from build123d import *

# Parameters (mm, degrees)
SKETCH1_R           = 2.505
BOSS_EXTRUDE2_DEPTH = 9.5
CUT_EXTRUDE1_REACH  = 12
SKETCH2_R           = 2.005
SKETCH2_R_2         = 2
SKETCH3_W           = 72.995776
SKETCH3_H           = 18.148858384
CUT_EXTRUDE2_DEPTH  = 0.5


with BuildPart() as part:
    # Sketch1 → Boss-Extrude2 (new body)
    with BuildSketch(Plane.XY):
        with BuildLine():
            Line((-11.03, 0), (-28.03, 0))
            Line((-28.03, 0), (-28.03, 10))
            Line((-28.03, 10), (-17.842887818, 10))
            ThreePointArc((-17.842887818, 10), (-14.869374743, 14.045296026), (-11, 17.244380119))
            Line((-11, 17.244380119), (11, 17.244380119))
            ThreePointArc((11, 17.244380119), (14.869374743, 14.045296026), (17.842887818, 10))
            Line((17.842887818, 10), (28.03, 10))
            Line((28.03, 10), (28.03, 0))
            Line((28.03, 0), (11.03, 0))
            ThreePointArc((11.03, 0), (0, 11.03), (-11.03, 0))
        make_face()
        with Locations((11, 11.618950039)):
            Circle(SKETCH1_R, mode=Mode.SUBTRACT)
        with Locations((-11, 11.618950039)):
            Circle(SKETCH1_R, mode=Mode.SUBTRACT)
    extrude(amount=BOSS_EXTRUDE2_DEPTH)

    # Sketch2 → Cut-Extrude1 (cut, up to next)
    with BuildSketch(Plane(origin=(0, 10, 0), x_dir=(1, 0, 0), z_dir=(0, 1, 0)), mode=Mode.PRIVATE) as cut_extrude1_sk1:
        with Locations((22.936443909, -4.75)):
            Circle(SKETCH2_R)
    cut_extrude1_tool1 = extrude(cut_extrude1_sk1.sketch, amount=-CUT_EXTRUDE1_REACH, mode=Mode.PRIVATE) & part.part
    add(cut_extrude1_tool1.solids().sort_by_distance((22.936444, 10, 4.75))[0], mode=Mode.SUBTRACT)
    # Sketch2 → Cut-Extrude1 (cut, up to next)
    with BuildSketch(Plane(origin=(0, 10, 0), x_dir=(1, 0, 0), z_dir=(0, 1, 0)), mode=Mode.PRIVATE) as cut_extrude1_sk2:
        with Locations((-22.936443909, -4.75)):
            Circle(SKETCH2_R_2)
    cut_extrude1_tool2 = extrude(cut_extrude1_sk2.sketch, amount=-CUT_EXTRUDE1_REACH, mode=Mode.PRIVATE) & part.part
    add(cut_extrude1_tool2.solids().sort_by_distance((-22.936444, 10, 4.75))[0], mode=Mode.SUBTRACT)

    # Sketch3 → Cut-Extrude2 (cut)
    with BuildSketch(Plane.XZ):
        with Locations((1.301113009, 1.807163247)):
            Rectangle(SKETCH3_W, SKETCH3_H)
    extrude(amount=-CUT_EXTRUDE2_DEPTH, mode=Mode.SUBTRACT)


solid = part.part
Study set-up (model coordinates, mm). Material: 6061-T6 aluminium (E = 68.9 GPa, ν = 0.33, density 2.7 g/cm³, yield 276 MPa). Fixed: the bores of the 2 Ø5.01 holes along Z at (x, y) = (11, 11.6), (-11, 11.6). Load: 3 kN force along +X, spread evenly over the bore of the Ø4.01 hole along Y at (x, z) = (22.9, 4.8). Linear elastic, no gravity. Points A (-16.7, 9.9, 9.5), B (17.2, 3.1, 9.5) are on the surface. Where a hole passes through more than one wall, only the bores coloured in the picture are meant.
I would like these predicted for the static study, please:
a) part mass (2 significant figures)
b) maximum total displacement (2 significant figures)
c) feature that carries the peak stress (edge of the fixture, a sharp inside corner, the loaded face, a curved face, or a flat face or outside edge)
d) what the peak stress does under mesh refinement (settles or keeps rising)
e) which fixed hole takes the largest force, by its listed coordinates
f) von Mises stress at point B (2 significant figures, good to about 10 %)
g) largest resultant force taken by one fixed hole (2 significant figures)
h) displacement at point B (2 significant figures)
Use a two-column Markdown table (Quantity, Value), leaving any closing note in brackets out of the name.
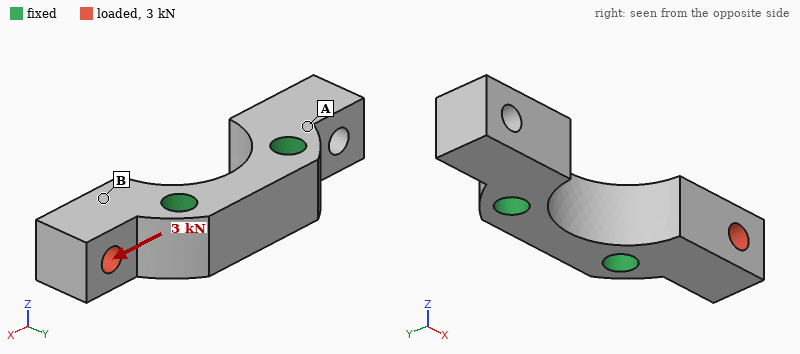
| Quantity | Value |
|---|---|
| part mass | 13 g |
| maximum total displacement | 46 µm |
| feature that carries the peak stress | edge of the fixture |
| what the peak stress does under mesh refinement | keeps rising |
| which fixed hole takes the largest force, by its listed coordinates | (11, 11.6) |
| von Mises stress at point B | 39 MPa |
| largest resultant force taken by one fixed hole | 3.0 kN |
| displacement at point B | 22 µm |
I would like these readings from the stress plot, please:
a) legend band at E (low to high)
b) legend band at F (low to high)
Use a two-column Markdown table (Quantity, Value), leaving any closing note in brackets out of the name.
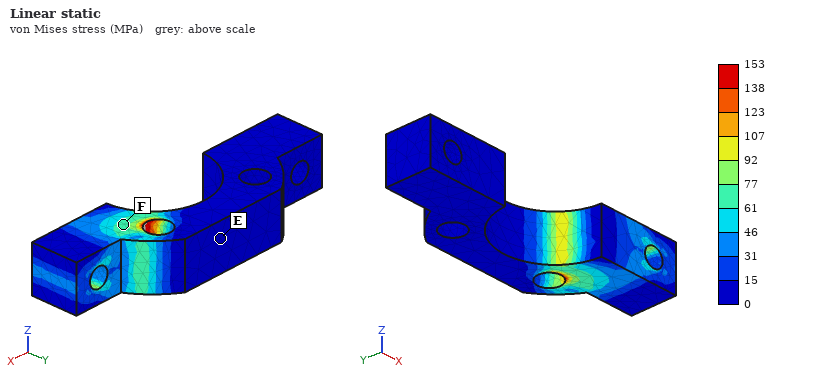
| Quantity | Value |
|---|---|
| legend band at E | 0 to 15 MPa |
| legend band at F | 61 to 77 MPa |
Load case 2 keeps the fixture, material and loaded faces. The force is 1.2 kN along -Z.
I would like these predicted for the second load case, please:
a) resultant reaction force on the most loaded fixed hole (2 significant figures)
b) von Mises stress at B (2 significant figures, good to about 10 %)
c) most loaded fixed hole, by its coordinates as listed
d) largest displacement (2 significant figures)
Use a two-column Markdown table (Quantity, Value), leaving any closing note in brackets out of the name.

| Quantity | Value |
|---|---|
| resultant reaction force on the most loaded fixed hole | 1.2 kN |
| von Mises stress at B | 34 MPa |
| most loaded fixed hole, by its coordinates as listed | (11, 11.6) |
| largest displacement | 43 µm |
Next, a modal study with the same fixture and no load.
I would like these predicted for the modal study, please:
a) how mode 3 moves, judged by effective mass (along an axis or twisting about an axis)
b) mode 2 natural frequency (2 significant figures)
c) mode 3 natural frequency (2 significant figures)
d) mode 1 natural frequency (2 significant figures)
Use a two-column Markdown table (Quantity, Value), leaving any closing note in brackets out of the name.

| Quantity | Value |
|---|---|
| how mode 3 moves, judged by effective mass | along Z |
| mode 2 natural frequency | 19 kHz |
| mode 3 natural frequency | 21 kHz |
| mode 1 natural frequency | 19 kHz |
